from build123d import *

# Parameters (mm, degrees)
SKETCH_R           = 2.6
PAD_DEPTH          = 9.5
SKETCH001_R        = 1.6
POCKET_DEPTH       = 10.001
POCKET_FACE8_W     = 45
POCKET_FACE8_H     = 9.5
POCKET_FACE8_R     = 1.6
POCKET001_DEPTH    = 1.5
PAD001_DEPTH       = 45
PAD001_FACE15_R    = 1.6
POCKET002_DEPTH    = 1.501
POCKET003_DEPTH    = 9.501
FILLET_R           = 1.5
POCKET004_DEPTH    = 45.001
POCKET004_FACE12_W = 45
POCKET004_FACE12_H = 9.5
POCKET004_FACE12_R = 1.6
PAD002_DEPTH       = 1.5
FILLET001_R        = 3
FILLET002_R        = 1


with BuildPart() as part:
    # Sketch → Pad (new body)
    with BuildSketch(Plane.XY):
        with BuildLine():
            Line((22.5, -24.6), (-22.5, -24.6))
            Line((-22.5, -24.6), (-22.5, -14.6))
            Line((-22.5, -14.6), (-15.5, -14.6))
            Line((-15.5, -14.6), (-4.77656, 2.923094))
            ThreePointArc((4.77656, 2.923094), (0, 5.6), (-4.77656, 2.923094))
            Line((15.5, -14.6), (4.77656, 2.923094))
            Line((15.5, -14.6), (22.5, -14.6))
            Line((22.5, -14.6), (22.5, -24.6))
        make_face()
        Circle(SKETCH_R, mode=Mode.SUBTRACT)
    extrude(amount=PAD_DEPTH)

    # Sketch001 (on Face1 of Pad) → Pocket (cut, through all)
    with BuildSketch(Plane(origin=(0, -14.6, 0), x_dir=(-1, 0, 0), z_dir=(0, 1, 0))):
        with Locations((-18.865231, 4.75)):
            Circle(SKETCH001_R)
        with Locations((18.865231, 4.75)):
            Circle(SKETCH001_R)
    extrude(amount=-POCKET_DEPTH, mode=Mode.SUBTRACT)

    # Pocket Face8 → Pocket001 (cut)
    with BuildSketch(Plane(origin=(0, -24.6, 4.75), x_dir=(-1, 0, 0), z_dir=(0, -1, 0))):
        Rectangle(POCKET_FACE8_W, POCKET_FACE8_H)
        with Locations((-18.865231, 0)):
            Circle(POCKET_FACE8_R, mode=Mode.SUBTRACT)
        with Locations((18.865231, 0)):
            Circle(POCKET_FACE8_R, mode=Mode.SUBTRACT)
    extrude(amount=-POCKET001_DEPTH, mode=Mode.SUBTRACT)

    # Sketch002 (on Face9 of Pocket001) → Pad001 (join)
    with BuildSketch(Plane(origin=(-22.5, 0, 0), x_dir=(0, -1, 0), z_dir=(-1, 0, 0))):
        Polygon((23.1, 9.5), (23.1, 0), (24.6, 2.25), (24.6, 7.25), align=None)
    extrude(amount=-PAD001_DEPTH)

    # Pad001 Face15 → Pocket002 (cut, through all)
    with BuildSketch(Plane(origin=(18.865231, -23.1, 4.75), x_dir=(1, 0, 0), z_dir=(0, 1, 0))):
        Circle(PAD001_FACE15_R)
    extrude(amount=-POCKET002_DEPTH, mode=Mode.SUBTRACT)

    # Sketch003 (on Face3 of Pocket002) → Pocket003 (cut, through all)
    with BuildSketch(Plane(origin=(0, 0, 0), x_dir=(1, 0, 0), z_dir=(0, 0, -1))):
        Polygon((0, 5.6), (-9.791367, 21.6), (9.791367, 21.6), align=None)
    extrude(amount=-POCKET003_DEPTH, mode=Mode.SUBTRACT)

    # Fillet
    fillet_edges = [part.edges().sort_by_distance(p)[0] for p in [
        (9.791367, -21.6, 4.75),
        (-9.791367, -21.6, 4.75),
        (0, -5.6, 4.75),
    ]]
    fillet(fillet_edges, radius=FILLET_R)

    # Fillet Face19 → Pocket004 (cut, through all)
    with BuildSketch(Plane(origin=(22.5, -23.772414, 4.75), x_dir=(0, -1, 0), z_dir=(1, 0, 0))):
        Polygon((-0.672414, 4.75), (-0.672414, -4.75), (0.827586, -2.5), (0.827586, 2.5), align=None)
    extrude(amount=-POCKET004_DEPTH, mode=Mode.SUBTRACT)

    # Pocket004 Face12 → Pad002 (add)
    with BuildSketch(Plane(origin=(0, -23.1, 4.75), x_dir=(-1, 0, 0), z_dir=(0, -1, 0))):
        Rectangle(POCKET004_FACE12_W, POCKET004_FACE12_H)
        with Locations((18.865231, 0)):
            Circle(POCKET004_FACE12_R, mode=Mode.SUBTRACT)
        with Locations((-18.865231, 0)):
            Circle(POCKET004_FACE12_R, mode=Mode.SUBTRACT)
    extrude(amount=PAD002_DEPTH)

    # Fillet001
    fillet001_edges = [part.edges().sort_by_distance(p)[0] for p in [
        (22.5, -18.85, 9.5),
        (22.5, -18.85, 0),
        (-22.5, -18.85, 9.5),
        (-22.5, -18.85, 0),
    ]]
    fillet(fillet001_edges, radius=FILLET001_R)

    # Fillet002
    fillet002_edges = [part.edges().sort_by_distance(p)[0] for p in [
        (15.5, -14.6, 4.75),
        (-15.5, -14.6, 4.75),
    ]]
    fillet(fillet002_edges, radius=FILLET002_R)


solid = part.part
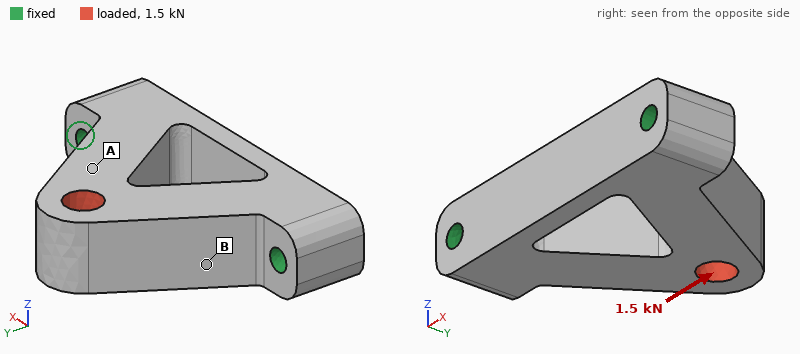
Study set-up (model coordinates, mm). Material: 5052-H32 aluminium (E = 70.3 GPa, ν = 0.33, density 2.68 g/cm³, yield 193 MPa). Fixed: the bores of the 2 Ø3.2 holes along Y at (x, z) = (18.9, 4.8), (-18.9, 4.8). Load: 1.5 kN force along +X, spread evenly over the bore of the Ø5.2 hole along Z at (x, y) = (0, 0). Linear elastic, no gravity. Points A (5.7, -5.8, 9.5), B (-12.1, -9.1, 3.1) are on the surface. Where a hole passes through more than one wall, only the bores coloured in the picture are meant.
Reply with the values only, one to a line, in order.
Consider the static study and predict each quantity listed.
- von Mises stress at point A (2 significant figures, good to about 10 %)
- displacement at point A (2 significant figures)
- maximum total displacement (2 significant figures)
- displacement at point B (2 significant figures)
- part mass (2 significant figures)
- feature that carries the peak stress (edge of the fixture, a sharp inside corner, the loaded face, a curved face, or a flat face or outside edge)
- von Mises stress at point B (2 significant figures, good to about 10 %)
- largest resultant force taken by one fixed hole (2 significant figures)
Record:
9.6 MPa
6.5 µm
14 µm
5.1 µm
16 g
a curved face
24 MPa
1.1 kN
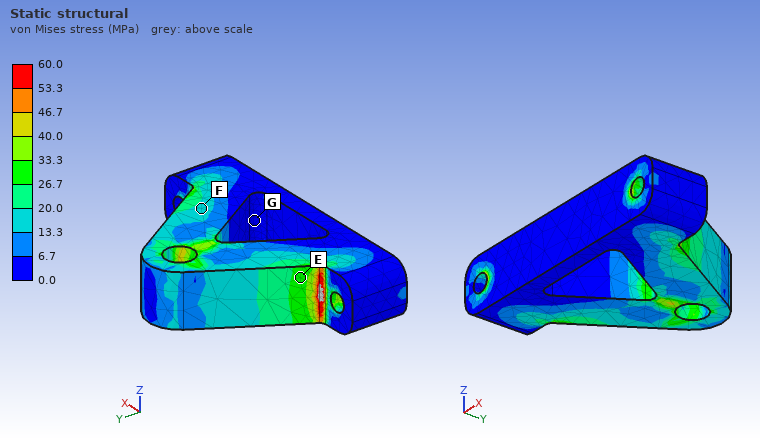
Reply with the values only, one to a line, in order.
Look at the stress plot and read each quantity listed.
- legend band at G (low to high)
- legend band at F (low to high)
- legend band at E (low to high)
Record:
0.0 to 6.7 MPa
13.3 to 20.0 MPa
26.7 to 33.3 MPa
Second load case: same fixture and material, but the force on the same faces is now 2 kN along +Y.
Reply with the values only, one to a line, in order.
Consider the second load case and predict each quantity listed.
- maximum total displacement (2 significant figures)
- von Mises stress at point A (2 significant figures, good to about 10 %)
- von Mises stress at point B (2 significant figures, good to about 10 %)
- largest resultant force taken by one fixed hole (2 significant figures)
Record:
9.5 µm
16 MPa
19 MPa
1.1 kN
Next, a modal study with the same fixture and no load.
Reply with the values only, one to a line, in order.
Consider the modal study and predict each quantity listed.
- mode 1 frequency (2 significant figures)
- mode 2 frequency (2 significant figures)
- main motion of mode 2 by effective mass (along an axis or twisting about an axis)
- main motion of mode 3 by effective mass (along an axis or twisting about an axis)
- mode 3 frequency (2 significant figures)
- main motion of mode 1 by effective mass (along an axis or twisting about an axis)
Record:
9300 Hz
26 kHz
along Z
along Y
27 kHz
along Z
